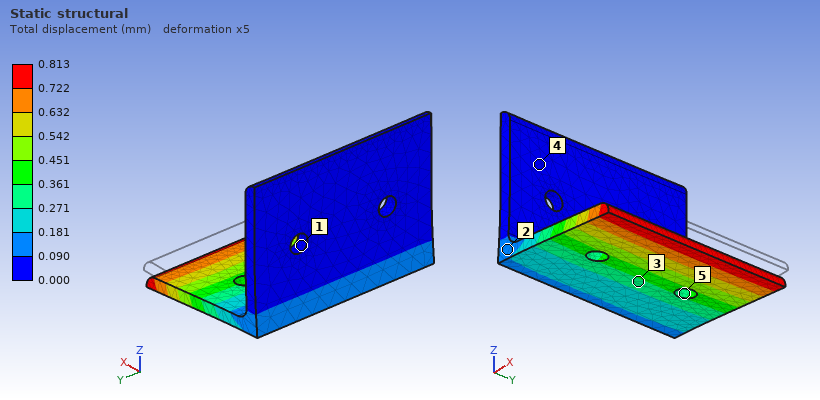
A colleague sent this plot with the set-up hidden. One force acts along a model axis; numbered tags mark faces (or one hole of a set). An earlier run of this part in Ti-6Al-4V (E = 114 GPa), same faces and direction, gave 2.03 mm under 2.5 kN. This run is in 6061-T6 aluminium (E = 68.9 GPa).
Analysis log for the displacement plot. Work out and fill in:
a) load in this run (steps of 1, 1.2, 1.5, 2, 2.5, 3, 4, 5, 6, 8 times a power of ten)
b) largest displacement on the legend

600 N
0.813 mm
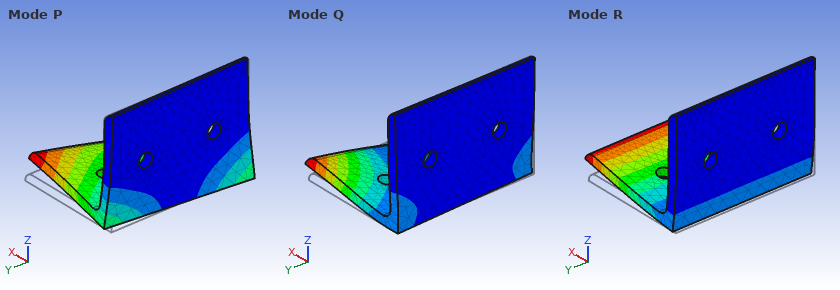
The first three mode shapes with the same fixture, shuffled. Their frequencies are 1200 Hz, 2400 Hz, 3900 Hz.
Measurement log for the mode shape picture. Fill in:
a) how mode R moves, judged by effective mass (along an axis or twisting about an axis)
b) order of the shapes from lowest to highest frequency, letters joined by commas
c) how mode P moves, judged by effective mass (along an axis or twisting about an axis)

along Z
R, P, Q
along Y
